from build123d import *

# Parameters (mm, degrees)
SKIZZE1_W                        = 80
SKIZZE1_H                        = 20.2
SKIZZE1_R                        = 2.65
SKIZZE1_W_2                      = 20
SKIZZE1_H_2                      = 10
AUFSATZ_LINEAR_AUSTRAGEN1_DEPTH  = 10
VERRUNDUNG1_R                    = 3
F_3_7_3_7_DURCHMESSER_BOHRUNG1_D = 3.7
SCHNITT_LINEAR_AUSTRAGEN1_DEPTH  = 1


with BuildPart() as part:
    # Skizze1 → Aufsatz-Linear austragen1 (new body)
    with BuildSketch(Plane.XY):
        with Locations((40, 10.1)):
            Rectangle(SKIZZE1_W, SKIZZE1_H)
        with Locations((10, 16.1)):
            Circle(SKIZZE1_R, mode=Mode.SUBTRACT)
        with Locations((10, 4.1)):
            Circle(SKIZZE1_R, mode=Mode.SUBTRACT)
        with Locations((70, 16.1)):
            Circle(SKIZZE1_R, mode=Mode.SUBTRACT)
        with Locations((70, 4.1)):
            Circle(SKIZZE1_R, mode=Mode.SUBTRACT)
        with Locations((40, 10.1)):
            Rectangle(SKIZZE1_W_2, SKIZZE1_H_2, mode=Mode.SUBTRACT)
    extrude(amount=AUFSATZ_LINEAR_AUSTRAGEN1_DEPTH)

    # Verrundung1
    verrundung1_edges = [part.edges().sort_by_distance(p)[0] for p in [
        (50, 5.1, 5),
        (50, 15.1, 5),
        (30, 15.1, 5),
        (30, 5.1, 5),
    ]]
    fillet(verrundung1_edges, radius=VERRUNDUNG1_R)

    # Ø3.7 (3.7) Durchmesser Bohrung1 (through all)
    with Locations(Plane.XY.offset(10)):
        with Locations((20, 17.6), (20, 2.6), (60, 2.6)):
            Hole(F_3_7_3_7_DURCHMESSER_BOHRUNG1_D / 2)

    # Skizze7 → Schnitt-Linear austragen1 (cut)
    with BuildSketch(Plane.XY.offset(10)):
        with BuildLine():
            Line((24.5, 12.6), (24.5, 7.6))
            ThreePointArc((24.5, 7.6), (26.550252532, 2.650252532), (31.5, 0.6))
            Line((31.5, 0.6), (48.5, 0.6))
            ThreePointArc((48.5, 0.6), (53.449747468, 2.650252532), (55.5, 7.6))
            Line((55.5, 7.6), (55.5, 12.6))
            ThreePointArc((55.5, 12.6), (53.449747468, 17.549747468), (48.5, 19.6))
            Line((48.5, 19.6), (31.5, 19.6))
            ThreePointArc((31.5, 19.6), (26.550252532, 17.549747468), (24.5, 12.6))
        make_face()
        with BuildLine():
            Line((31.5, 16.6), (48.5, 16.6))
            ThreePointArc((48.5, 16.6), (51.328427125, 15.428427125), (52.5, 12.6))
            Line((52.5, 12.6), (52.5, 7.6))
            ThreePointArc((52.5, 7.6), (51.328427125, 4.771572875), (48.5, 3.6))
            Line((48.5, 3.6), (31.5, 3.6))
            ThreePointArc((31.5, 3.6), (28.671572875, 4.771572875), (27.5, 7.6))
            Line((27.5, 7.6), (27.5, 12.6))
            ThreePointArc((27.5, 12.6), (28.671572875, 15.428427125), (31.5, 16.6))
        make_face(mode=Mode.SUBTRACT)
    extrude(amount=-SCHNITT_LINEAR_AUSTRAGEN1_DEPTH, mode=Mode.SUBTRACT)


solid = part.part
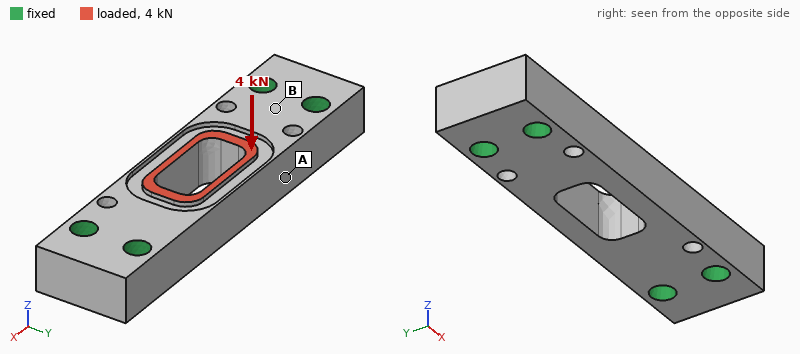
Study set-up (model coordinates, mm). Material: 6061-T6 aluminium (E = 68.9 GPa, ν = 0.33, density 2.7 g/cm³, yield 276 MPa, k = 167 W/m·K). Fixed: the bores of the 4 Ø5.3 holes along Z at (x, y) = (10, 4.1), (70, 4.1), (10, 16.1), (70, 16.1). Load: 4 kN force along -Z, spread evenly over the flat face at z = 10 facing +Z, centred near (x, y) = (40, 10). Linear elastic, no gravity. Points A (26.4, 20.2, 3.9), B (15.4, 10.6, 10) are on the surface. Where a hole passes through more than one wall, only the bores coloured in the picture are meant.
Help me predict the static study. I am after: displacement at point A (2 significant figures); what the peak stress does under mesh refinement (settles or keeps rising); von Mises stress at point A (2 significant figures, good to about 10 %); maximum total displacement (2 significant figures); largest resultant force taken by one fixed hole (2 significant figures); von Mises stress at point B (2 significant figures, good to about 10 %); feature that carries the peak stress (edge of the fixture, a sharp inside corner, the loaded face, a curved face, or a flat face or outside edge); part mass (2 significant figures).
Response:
27 µm
keeps rising
29 MPa
52 µm
1.0 kN
56 MPa
edge of the fixture
35 g
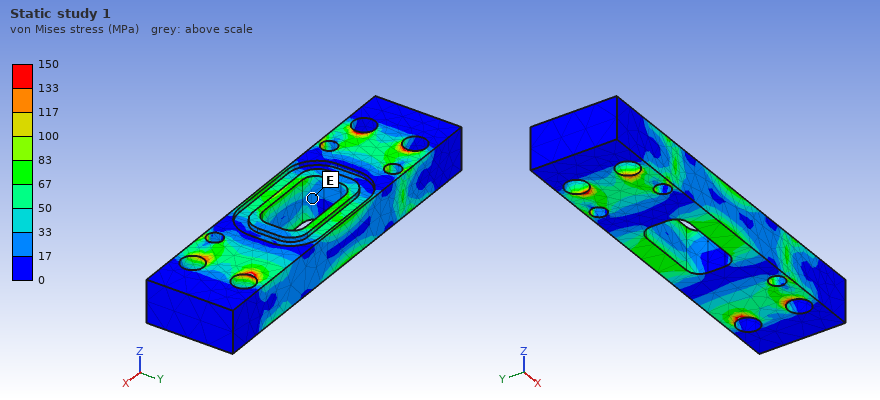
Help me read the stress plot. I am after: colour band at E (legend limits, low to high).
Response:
17 to 33 MPa
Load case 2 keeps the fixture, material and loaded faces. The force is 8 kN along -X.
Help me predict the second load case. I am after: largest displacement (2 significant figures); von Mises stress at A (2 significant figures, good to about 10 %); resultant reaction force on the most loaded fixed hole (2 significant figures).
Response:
21 µm
15 MPa
2.3 kN
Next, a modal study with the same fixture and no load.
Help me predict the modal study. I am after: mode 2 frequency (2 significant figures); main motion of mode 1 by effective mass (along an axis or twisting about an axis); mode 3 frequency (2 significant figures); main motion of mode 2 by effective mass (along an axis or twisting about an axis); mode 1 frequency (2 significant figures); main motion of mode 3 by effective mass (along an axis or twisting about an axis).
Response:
21 kHz
along Z
22 kHz
twisting about X
15 kHz
along Y
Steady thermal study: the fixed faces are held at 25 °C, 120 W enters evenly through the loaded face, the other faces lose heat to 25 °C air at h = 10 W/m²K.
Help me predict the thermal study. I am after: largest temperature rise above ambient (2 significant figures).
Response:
61 K
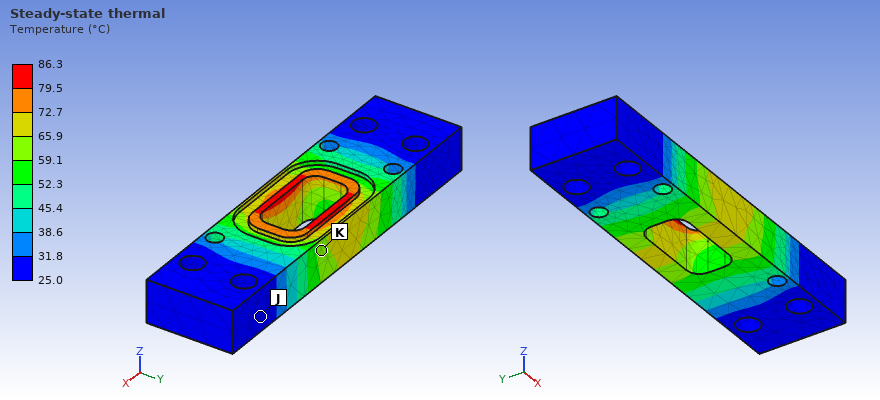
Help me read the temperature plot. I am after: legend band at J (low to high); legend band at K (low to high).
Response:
25.0 to 31.8 °C
59.1 to 65.9 °C
